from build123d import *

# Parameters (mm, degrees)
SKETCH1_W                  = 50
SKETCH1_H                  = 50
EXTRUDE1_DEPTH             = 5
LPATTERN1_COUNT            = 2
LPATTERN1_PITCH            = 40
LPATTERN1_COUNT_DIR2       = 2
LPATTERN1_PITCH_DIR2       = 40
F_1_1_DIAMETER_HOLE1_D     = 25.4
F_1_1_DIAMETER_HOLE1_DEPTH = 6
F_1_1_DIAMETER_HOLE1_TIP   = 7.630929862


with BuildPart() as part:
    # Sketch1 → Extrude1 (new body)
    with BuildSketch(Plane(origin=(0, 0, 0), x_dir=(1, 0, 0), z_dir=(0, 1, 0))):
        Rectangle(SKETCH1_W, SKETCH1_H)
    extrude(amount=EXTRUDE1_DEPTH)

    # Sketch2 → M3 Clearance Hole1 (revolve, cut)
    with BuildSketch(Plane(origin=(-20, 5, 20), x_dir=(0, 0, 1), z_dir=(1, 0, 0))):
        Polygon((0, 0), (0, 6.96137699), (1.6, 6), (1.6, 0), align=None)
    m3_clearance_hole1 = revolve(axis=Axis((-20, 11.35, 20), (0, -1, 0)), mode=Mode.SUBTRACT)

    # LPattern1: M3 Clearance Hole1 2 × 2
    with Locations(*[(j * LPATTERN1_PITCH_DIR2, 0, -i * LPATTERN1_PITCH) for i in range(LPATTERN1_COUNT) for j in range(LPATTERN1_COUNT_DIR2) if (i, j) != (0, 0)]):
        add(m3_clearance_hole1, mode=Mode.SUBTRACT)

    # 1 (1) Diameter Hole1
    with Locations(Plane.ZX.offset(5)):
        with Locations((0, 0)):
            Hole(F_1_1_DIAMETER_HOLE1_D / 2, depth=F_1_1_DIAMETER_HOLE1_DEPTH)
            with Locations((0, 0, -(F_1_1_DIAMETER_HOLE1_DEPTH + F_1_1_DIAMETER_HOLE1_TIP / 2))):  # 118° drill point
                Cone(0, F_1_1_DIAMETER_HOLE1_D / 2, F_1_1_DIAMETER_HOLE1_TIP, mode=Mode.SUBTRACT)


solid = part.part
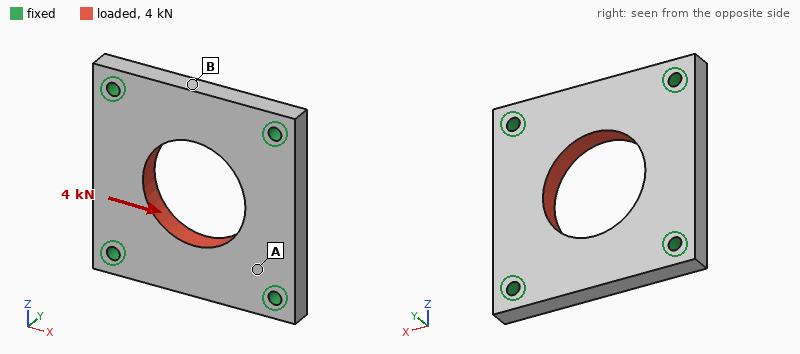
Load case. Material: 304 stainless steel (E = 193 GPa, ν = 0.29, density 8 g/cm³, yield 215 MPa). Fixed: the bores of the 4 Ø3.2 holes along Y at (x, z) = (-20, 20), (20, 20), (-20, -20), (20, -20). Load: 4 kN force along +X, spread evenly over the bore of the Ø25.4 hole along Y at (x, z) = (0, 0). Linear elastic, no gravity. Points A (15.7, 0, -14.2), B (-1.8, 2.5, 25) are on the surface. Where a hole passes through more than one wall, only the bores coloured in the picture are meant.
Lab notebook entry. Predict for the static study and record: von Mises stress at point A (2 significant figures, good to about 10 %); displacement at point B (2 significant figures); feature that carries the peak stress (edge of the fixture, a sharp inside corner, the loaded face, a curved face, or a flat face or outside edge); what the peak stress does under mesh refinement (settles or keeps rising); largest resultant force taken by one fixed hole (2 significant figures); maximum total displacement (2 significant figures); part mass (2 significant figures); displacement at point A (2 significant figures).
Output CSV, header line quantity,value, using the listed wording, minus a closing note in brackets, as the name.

quantity,value
von Mises stress at point A,16 MPa
displacement at point B,0.98 µm
feature that carries the peak stress,edge of the fixture
what the peak stress does under mesh refinement,keeps rising
largest resultant force taken by one fixed hole,1.1 kN
maximum total displacement,3.1 µm
part mass,78 g
displacement at point A,1.1 µm
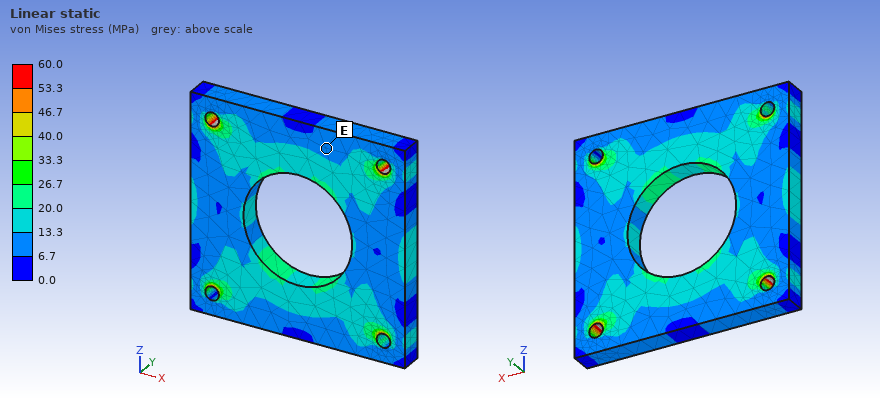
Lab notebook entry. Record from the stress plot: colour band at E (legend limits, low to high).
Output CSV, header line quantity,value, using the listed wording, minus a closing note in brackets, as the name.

quantity,value
colour band at E,6.7 to 13.3 MPa
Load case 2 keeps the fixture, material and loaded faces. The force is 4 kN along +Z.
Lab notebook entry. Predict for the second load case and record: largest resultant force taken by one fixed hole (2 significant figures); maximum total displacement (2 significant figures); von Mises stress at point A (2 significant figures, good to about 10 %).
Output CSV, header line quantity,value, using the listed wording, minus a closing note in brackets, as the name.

quantity,value
largest resultant force taken by one fixed hole,1.1 kN
maximum total displacement,3.1 µm
von Mises stress at point A,16 MPa
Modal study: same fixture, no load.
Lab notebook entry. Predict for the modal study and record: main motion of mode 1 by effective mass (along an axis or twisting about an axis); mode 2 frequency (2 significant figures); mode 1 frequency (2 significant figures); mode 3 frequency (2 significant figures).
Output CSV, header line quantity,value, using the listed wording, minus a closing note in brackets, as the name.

quantity,value
main motion of mode 1 by effective mass,along Y
mode 2 frequency,15 kHz
mode 1 frequency,12 kHz
mode 3 frequency,15 kHz
